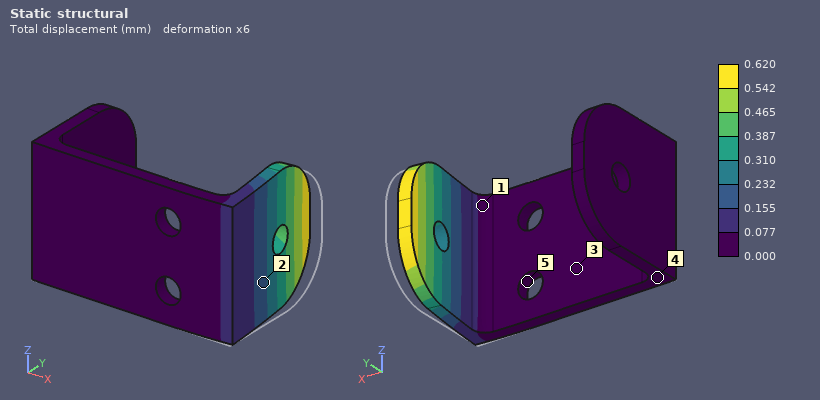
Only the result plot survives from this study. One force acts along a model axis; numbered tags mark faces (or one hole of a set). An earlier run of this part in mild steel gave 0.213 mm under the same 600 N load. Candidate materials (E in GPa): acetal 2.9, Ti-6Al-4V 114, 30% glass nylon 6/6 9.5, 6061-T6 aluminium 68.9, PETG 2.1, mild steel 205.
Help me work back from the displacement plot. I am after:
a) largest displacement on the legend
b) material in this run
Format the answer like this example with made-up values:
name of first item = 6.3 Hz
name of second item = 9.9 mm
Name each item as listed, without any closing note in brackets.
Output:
largest displacement on the legend = 0.620 mm
material in this run = 6061-T6 aluminium
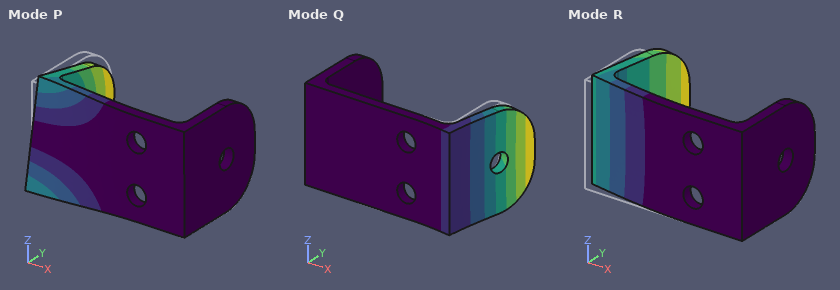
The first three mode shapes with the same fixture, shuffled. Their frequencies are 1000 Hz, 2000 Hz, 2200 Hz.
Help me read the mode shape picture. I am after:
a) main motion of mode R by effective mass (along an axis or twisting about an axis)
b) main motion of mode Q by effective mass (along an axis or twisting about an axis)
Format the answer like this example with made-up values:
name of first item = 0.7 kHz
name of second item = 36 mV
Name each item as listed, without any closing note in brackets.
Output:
main motion of mode R by effective mass = along Y
main motion of mode Q by effective mass = along X
